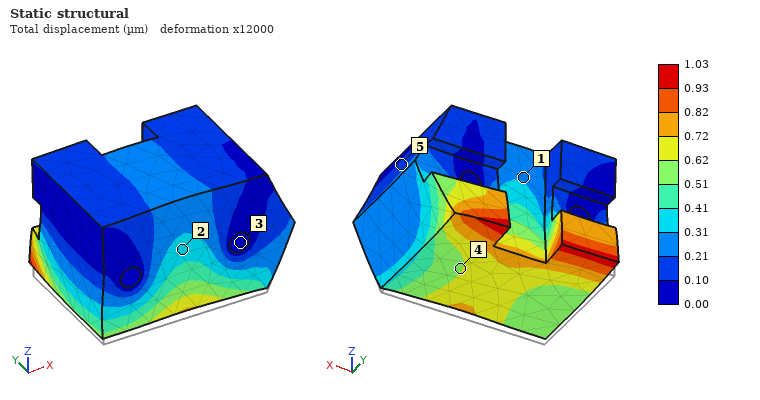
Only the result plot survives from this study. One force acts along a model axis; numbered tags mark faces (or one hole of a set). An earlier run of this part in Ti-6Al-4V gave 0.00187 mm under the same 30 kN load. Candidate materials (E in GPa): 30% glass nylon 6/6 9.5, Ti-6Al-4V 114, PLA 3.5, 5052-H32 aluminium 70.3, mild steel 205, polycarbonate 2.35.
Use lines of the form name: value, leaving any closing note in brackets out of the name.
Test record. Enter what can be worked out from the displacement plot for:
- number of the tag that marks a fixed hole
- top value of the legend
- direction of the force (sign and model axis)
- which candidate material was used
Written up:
number of the tag that marks a fixed hole: 3
top value of the legend: 1.03 µm
direction of the force: +Z
which candidate material was used: mild steel
